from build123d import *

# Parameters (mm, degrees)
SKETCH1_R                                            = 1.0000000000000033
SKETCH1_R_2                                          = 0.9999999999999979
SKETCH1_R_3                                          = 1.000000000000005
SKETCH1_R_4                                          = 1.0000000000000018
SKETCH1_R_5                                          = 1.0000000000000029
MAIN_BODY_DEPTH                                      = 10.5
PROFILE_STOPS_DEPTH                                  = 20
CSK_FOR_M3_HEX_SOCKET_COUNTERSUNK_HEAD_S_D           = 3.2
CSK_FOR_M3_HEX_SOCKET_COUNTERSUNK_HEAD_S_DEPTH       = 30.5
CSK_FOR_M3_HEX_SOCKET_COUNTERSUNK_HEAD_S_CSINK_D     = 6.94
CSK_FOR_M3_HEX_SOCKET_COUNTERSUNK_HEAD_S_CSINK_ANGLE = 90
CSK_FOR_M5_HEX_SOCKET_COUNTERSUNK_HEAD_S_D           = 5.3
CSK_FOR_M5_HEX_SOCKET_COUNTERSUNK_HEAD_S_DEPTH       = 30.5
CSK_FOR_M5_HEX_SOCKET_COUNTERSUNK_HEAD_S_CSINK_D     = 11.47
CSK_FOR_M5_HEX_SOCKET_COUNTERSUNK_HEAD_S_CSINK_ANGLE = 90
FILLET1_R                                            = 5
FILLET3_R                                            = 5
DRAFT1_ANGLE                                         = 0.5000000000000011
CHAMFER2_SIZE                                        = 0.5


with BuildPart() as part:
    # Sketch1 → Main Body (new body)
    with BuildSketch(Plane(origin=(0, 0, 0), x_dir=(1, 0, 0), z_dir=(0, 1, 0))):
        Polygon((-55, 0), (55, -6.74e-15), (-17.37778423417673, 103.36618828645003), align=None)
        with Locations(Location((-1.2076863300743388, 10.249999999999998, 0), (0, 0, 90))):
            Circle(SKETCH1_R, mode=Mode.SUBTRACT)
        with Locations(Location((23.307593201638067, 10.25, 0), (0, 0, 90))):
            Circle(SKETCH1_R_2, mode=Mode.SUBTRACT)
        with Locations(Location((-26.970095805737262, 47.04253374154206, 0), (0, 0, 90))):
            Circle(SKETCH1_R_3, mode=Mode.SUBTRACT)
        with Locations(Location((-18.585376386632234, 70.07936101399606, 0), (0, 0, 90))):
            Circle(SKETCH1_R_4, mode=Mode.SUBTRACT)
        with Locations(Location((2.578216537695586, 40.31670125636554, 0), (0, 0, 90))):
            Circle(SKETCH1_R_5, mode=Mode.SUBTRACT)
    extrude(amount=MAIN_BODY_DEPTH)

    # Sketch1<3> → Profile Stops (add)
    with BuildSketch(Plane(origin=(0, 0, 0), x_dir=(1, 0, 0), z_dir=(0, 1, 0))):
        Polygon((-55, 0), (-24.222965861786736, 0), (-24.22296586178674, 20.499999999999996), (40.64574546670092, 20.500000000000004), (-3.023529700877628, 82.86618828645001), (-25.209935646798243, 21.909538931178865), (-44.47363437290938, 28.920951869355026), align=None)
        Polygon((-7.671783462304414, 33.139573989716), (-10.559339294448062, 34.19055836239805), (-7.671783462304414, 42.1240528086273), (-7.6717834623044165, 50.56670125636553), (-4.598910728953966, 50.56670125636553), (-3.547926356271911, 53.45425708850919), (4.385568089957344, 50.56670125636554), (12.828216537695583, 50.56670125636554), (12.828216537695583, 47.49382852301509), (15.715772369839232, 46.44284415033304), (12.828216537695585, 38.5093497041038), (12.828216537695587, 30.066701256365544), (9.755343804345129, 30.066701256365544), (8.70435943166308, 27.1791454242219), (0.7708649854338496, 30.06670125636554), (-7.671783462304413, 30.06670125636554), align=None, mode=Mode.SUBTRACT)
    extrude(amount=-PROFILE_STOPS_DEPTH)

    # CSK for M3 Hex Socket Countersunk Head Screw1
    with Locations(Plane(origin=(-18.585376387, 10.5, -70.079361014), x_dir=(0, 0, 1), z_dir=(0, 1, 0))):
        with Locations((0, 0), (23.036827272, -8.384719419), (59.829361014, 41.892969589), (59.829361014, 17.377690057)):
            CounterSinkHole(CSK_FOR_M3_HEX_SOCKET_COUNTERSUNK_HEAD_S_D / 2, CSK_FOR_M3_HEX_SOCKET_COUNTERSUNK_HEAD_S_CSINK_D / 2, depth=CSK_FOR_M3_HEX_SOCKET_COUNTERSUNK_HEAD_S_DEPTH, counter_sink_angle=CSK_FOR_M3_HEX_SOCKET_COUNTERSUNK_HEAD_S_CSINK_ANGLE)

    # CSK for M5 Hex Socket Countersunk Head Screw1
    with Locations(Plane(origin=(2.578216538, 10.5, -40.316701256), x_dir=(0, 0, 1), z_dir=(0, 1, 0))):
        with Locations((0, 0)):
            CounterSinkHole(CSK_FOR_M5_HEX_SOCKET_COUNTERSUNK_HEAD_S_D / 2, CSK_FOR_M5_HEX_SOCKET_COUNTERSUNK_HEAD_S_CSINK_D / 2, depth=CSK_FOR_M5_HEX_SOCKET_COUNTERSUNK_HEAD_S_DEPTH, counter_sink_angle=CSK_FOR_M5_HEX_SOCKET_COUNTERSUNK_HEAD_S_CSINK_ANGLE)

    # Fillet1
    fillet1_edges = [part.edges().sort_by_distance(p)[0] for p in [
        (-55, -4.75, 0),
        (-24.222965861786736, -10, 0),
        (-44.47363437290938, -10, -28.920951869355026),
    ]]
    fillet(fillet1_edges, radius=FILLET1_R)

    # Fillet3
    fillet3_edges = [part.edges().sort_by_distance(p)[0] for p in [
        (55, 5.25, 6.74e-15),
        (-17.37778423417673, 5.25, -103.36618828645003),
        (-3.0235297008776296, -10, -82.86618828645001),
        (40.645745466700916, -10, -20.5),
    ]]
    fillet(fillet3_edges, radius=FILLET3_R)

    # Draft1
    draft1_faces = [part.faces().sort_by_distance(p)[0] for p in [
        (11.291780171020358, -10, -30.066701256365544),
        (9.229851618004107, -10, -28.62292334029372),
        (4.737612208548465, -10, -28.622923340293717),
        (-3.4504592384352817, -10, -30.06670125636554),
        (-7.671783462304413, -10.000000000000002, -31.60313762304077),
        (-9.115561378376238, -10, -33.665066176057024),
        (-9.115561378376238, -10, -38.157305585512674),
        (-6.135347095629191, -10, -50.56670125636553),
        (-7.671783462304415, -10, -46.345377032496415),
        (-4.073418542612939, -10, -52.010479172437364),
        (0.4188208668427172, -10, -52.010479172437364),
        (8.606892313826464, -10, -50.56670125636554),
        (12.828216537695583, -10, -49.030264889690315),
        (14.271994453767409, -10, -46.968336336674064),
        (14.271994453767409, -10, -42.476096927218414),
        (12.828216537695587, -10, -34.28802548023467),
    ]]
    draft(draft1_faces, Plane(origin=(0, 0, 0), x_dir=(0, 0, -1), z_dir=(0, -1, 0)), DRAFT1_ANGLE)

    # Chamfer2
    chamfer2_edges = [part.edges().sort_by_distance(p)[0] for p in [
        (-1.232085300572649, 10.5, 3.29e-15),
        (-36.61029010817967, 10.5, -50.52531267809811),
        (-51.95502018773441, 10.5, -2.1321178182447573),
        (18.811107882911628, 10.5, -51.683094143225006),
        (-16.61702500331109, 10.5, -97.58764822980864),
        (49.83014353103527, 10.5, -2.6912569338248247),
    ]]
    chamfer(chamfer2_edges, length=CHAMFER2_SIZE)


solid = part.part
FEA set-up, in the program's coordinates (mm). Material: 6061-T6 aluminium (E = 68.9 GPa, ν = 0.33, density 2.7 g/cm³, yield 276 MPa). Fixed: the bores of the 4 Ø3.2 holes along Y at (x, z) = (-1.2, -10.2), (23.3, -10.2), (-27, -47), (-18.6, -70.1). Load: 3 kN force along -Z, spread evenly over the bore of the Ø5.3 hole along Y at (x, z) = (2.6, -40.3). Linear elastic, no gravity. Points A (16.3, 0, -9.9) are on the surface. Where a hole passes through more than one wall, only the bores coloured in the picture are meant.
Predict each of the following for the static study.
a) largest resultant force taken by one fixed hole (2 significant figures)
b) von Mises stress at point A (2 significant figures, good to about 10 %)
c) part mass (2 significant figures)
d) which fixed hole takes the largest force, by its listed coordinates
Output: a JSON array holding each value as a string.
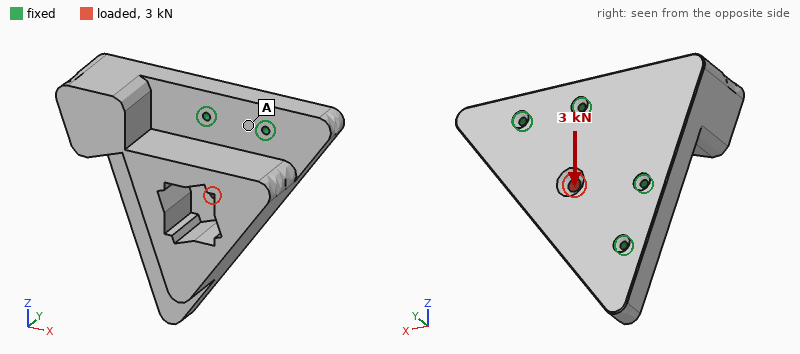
["1.1 kN", "2.5 MPa", "280 g", "(-1.2, -10.2)"]
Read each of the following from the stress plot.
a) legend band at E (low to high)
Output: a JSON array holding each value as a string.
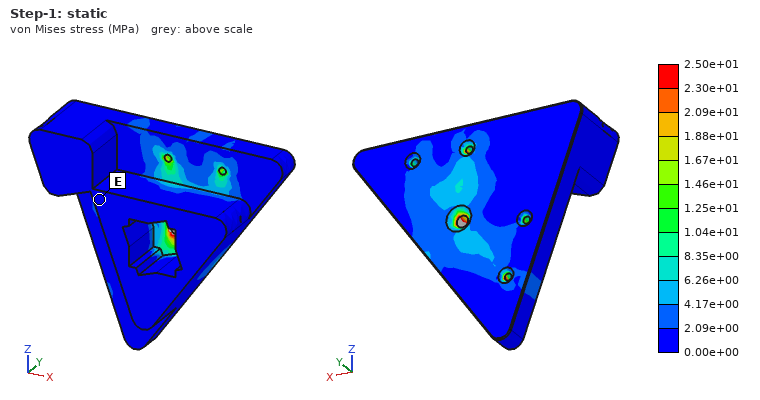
["0.00e+00 to 2.09e+00 MPa"]
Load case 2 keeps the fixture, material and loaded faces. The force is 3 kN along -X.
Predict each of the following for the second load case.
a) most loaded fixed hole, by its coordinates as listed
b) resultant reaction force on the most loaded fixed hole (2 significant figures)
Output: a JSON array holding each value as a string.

["(-27, -47)", "1.3 kN"]
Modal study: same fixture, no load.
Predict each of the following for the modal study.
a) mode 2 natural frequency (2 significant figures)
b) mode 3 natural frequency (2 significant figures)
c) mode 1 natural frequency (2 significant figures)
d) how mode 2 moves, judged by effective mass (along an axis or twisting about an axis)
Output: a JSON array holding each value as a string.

["6800 Hz", "8700 Hz", "4000 Hz", "along Y"]
